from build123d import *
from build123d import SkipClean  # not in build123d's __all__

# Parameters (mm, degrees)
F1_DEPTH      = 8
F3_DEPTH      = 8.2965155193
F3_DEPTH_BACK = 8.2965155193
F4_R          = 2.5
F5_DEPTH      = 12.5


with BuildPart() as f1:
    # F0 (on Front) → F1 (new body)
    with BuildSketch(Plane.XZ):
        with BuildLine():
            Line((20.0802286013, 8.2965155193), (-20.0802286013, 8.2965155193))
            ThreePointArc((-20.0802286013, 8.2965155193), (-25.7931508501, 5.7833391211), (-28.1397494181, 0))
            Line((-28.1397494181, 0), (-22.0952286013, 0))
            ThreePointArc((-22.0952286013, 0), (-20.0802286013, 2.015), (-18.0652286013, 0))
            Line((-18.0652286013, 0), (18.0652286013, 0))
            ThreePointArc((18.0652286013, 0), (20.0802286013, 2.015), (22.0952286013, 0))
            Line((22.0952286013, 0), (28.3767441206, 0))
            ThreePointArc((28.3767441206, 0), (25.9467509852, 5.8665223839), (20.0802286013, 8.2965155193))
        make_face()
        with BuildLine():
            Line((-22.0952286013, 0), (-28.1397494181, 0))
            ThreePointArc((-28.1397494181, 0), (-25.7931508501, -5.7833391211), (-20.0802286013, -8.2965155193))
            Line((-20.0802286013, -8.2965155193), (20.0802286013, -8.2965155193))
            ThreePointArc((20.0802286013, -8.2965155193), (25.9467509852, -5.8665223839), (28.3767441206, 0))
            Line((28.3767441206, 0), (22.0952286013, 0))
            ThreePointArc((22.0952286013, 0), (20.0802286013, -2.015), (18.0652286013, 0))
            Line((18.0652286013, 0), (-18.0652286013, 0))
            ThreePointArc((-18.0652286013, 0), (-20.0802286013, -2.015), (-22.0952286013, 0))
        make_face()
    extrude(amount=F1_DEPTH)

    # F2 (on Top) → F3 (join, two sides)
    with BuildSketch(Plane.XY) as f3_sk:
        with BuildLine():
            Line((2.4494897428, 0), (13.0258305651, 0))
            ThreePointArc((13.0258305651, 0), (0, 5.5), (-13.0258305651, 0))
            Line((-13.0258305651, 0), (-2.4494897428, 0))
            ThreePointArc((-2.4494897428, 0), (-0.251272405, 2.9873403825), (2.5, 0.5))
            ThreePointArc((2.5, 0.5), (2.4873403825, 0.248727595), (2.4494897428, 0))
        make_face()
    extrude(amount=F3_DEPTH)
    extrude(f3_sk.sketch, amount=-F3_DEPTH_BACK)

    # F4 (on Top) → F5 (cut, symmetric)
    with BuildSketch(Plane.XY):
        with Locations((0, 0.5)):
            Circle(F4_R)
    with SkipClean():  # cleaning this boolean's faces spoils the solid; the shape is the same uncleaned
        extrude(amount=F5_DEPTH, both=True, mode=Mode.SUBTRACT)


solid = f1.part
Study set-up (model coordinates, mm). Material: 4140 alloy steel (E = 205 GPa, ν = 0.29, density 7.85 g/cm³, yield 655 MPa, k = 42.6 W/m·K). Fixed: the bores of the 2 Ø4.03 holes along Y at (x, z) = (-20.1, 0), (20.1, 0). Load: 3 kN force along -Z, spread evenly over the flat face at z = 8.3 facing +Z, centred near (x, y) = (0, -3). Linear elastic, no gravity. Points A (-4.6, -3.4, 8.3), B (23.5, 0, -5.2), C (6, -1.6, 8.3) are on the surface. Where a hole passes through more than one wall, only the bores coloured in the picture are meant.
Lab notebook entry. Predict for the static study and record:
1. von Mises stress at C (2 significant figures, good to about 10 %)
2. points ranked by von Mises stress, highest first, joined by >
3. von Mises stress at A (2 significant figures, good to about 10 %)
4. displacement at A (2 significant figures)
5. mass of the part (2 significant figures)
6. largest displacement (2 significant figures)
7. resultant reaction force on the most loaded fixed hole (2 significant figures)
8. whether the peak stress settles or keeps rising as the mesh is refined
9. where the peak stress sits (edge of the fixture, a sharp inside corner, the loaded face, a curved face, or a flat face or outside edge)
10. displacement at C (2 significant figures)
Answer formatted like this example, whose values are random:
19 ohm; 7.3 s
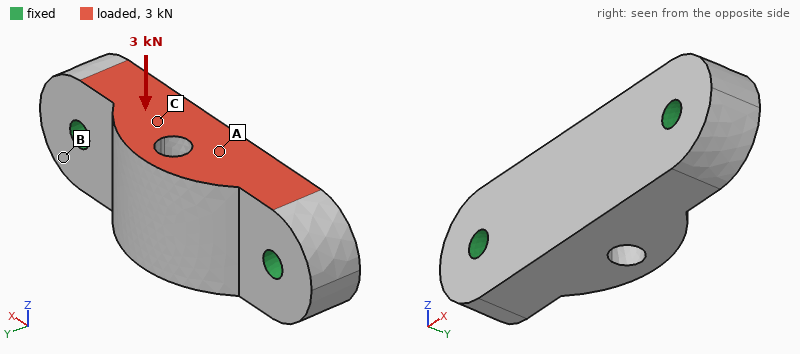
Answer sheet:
17 MPa; A > C > B; 25 MPa; 3.7 µm; 64 g; 5.4 µm; 1.5 kN; keeps rising; edge of the fixture; 3.9 µm
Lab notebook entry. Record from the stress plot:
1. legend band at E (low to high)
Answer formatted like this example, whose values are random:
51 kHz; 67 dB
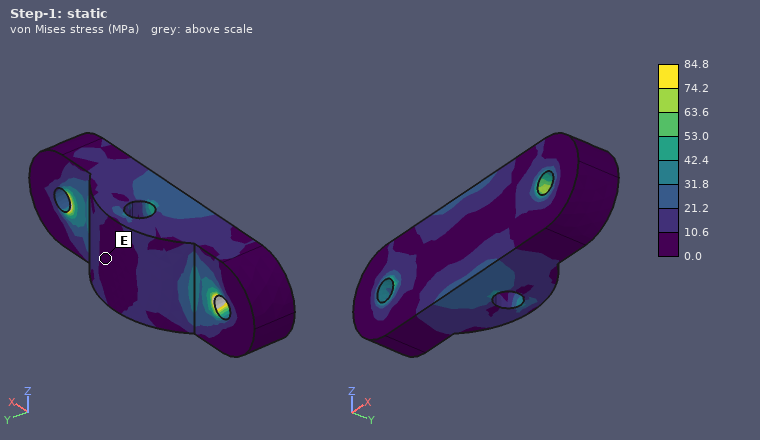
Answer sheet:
0.0 to 10.6 MPa
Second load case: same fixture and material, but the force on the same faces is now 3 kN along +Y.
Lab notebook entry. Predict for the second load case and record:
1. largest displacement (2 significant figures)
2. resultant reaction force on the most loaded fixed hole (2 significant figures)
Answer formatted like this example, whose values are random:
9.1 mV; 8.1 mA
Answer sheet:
12 µm; 1.5 kN
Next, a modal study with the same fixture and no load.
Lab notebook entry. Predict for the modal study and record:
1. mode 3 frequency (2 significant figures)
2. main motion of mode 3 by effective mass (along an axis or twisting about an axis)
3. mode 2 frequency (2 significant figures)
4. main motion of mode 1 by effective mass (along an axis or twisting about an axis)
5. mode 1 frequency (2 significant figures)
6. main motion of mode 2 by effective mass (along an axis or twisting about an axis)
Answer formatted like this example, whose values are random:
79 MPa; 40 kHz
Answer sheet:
26 kHz; along Z; 21 kHz; along Z; 19 kHz; along Y
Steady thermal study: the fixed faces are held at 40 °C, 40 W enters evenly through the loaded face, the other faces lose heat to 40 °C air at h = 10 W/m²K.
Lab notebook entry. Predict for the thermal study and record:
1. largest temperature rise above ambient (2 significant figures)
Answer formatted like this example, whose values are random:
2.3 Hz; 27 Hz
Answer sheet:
51 K
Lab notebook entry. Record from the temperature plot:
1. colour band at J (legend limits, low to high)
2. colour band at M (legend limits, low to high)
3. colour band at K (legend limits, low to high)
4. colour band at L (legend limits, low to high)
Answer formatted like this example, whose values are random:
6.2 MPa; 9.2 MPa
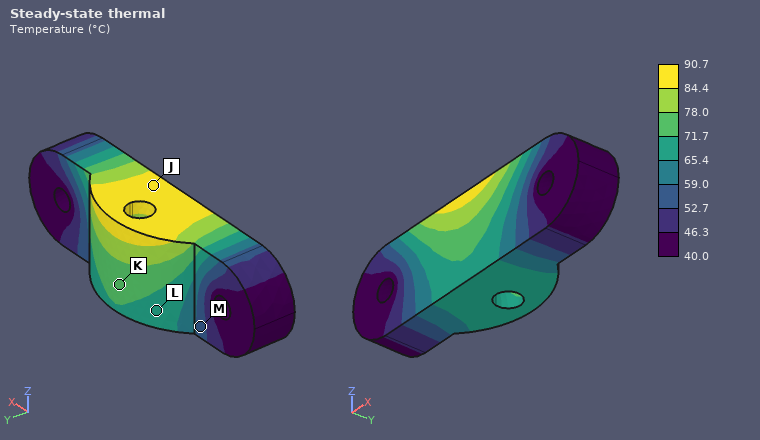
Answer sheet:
84.4 to 90.7 °C; 52.7 to 59.0 °C; 71.7 to 78.0 °C; 65.4 to 71.7 °C
